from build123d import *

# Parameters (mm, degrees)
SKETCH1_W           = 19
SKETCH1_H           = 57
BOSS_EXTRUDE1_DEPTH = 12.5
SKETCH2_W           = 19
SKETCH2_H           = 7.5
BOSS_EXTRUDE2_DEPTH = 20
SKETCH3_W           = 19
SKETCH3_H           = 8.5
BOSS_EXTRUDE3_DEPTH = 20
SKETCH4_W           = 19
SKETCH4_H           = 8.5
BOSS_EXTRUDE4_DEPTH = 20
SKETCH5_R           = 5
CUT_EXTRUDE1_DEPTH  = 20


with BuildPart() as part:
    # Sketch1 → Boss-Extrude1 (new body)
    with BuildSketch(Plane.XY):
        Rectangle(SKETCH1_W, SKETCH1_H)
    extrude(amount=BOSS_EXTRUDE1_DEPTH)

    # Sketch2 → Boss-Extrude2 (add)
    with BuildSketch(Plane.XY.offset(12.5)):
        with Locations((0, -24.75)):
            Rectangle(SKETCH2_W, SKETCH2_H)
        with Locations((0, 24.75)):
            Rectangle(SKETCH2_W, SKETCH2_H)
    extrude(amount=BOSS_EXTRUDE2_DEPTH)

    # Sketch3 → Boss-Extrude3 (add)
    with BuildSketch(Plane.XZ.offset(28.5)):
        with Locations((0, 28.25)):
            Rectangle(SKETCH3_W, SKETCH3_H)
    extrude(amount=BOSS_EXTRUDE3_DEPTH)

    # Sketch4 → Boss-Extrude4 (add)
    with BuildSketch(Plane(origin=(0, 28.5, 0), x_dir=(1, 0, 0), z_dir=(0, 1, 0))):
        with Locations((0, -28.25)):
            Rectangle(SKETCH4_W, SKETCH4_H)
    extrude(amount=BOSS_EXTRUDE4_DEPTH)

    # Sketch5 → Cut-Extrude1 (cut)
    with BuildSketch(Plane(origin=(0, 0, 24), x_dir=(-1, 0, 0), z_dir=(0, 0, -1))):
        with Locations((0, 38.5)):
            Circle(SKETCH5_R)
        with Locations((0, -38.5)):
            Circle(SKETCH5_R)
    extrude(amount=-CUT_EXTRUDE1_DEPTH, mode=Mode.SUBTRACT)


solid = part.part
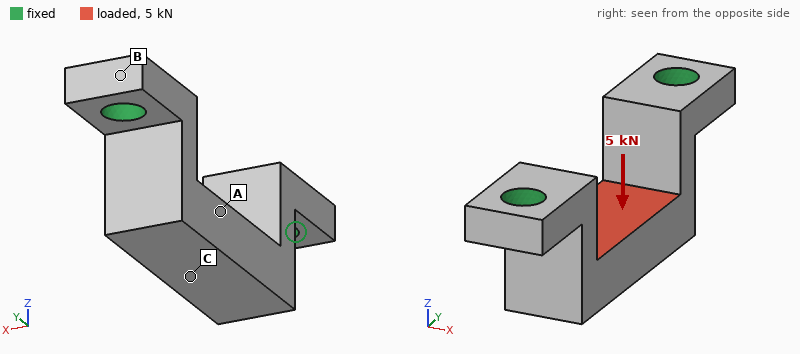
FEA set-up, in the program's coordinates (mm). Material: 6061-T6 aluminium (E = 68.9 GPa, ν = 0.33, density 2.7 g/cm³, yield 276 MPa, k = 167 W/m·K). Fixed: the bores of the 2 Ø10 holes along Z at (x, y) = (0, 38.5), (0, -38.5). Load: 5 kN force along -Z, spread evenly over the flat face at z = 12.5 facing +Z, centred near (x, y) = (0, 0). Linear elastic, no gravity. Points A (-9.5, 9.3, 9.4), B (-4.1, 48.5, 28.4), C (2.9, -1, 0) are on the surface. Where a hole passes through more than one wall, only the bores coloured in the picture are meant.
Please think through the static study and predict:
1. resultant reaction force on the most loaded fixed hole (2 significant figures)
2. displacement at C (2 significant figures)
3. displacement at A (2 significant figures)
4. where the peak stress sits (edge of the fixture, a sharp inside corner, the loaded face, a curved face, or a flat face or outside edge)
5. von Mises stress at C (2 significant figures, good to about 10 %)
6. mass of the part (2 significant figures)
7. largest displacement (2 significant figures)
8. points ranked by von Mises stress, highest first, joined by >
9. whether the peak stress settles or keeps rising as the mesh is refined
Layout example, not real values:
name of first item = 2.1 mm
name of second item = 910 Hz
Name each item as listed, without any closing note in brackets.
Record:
resultant reaction force on the most loaded fixed hole = 2.8 kN
displacement at C = 34 µm
displacement at A = 32 µm
where the peak stress sits = edge of the fixture
von Mises stress at C = 43 MPa
mass of the part = 66 g
largest displacement = 37 µm
points ranked by von Mises stress, highest first, joined by > = C > A > B
whether the peak stress settles or keeps rising as the mesh is refined = keeps rising
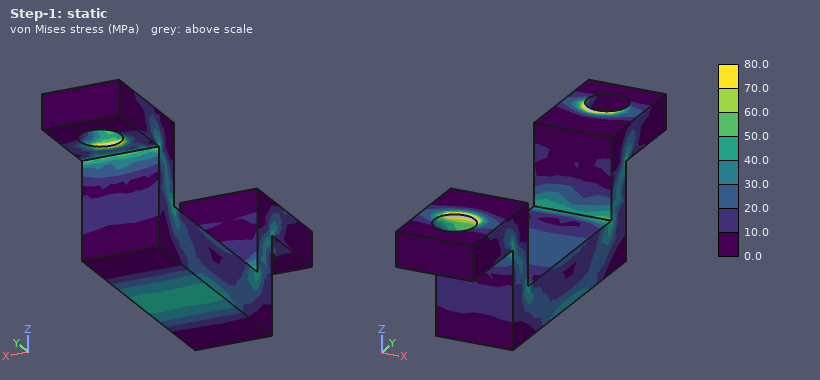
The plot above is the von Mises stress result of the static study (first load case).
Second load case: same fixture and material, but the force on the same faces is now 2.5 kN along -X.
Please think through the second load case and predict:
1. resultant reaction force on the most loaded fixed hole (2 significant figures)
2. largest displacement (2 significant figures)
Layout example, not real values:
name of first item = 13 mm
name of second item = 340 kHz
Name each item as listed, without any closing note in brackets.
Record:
resultant reaction force on the most loaded fixed hole = 1.3 kN
largest displacement = 79 µm
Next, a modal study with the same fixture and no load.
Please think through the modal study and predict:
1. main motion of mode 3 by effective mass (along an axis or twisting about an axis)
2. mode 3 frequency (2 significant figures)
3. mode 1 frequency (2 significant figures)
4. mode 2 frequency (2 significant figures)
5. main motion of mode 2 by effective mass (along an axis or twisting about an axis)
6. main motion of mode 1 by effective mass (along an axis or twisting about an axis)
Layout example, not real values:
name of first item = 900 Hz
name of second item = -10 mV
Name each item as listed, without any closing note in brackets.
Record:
main motion of mode 3 by effective mass = twisting about Z
mode 3 frequency = 8900 Hz
mode 1 frequency = 4300 Hz
mode 2 frequency = 7300 Hz
main motion of mode 2 by effective mass = along Y
main motion of mode 1 by effective mass = along X
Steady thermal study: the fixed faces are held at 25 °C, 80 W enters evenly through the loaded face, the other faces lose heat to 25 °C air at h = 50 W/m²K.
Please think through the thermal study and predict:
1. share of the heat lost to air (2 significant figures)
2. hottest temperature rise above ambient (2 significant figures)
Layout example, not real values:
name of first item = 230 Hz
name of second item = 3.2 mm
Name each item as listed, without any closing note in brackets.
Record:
share of the heat lost to air = 11 %
hottest temperature rise above ambient = 52 K
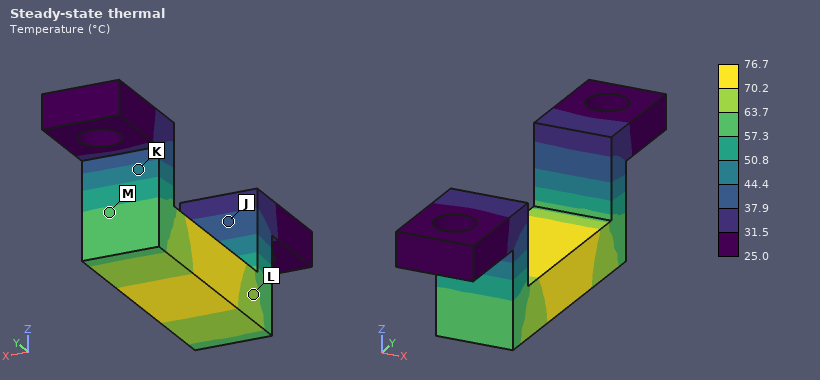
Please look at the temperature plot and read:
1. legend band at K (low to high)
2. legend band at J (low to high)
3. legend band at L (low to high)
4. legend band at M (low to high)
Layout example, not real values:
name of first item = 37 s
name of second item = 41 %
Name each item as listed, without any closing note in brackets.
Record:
legend band at K = 44.4 to 50.8 °C
legend band at J = 37.9 to 44.4 °C
legend band at L = 63.7 to 70.2 °C
legend band at M = 57.3 to 63.7 °C
